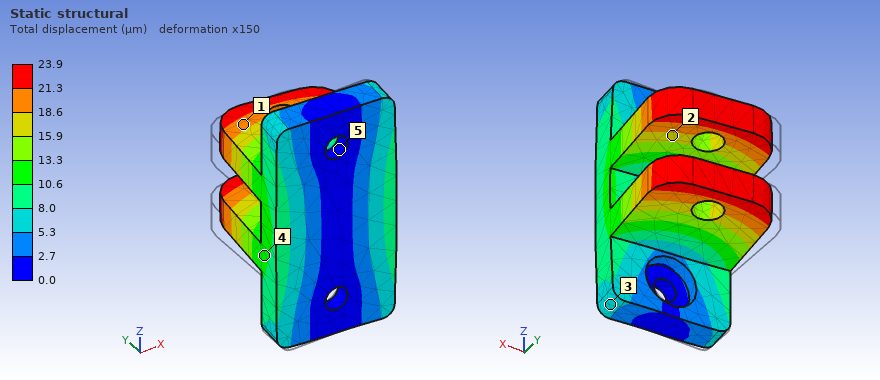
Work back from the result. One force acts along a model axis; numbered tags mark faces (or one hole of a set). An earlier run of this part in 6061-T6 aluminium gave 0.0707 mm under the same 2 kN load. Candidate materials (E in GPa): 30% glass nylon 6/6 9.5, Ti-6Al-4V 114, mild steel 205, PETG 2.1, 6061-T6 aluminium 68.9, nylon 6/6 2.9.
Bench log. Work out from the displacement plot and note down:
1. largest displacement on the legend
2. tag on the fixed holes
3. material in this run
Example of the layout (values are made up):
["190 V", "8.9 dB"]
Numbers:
["23.9 µm", "5", "mild steel"]
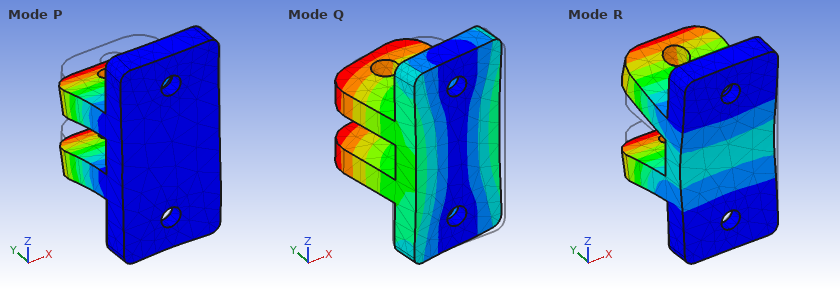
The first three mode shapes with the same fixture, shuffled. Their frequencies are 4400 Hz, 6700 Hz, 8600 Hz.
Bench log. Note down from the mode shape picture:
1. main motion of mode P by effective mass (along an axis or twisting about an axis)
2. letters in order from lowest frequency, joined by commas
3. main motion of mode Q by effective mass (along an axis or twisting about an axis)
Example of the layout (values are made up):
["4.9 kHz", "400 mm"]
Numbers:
["along Z", "Q, R, P", "along X"]
